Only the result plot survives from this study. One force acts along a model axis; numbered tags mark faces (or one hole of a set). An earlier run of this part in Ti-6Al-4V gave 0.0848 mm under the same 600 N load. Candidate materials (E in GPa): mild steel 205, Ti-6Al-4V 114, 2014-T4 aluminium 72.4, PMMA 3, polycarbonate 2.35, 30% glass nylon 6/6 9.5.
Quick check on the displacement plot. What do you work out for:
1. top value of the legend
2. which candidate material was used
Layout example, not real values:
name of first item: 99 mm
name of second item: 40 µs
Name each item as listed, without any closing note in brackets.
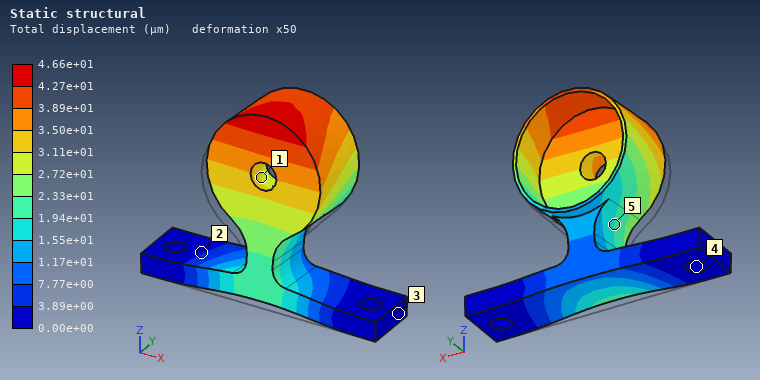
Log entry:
top value of the legend: 4.66e+01 µm
which candidate material was used: mild steel
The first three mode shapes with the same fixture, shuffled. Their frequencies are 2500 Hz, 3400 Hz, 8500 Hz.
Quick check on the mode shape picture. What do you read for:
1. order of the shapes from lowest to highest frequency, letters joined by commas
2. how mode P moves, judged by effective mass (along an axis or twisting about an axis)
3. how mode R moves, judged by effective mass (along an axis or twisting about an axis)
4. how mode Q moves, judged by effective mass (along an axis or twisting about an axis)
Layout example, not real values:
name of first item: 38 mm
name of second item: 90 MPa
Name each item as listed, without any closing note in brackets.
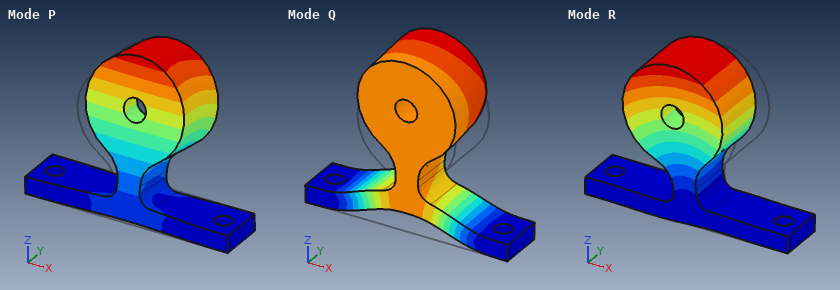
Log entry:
order of the shapes from lowest to highest frequency, letters joined by commas: P, R, Q
how mode P moves, judged by effective mass: along Y
how mode R moves, judged by effective mass: along X
how mode Q moves, judged by effective mass: along Z
